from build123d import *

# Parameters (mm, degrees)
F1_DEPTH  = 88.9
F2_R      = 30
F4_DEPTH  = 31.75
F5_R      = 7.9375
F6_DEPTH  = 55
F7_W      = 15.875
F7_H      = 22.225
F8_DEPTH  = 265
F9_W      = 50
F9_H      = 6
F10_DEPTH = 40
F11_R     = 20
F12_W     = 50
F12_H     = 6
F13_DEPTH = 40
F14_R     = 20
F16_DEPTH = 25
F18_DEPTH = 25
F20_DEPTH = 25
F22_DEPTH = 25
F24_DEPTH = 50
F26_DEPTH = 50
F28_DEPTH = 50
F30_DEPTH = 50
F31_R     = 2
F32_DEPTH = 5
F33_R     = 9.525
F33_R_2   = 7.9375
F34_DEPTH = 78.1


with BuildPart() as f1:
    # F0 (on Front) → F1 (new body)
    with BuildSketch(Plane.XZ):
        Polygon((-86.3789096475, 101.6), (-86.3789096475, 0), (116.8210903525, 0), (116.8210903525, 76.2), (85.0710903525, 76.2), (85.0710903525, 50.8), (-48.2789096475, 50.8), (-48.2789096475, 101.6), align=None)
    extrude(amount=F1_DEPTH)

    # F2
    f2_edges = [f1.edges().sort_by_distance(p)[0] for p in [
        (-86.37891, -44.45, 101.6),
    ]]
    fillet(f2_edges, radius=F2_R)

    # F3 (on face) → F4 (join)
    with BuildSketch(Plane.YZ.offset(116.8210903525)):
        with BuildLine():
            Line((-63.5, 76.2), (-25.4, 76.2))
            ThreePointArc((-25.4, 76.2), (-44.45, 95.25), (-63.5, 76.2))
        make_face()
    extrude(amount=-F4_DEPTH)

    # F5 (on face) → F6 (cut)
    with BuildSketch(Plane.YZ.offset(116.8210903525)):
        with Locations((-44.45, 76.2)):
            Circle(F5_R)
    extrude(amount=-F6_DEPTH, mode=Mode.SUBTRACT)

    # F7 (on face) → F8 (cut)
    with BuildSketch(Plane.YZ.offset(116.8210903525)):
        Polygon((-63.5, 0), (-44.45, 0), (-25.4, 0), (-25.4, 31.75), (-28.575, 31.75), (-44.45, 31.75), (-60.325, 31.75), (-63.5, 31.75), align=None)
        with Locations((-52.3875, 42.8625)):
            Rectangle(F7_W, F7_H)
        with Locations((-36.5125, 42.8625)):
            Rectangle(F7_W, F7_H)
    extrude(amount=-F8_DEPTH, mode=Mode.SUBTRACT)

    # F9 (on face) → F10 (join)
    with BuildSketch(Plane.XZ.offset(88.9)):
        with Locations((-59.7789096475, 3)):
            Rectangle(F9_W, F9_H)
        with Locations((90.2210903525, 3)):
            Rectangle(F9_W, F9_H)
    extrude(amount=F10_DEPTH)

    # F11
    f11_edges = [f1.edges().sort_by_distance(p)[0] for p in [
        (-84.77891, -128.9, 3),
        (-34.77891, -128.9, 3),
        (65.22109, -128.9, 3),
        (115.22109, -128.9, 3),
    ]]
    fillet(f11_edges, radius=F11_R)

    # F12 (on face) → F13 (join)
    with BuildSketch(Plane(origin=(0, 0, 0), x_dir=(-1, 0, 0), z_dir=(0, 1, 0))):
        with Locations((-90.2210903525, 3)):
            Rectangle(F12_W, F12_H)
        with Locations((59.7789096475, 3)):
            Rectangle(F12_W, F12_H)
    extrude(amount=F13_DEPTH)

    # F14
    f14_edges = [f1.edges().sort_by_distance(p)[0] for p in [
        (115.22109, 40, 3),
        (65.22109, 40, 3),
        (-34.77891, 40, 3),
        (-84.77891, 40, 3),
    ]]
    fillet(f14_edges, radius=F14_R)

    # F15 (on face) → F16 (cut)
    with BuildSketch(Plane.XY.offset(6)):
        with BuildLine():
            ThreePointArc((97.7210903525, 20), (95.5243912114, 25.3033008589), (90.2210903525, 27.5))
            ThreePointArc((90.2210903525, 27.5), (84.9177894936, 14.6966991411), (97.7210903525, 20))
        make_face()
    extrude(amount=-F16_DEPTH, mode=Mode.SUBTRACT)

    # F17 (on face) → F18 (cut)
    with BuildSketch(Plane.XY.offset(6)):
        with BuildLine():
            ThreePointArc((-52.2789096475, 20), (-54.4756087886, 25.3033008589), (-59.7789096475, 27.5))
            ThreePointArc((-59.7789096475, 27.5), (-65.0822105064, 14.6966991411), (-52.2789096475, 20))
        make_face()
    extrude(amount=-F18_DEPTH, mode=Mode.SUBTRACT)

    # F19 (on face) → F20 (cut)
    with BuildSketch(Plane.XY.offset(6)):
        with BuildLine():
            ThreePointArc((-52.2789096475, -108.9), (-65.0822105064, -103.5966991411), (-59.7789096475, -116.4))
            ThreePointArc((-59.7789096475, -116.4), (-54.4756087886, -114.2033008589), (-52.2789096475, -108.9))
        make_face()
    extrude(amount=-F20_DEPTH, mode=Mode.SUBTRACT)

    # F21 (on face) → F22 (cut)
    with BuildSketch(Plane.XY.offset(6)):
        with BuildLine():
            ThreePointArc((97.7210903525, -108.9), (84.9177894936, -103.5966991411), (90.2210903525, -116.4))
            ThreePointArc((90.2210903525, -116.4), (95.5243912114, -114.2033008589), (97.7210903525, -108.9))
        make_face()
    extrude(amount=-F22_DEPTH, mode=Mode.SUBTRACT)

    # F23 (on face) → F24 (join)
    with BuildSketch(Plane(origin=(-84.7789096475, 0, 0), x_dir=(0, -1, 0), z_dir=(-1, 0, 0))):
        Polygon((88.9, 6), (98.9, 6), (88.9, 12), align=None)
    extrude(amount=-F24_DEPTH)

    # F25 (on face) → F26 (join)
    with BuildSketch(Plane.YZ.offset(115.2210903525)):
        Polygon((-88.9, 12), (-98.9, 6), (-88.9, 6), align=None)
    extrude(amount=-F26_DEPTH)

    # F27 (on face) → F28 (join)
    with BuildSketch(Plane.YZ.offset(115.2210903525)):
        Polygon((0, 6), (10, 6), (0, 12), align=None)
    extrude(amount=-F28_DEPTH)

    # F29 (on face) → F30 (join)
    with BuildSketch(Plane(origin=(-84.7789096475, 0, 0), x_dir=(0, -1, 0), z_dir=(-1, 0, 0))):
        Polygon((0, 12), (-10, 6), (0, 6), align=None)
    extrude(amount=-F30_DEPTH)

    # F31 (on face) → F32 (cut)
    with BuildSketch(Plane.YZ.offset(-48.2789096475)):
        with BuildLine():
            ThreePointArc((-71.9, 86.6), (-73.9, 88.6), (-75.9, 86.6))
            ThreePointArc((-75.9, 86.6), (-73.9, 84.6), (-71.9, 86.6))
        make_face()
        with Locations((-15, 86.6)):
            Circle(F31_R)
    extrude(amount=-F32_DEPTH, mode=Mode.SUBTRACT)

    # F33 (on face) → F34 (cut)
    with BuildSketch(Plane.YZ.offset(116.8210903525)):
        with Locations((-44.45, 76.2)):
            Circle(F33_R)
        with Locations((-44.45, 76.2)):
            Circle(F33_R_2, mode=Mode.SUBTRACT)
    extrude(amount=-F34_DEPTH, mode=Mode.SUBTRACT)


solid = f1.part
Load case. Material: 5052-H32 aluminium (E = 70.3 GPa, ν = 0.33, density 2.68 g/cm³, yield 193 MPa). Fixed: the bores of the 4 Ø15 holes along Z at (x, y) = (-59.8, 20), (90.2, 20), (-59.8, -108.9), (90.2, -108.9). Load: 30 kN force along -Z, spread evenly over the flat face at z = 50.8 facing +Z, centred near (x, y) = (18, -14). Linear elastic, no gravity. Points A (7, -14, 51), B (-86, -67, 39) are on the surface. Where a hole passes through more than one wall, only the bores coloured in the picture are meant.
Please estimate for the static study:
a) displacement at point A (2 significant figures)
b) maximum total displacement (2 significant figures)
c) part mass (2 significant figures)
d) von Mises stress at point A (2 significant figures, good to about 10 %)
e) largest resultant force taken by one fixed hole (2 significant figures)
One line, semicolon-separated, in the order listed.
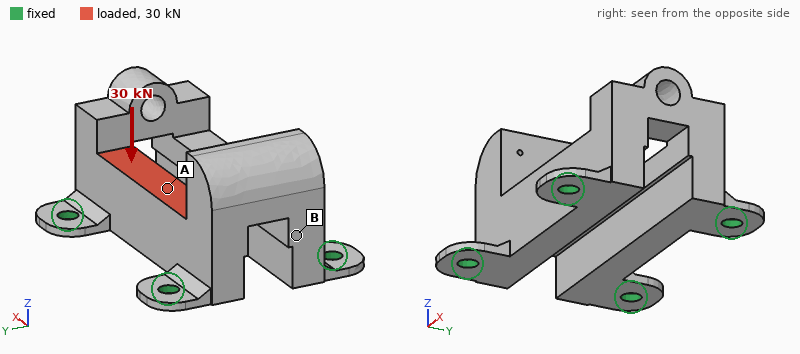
0.17 mm; 0.18 mm; 2.2 kg; 40 MPa; 13 kN
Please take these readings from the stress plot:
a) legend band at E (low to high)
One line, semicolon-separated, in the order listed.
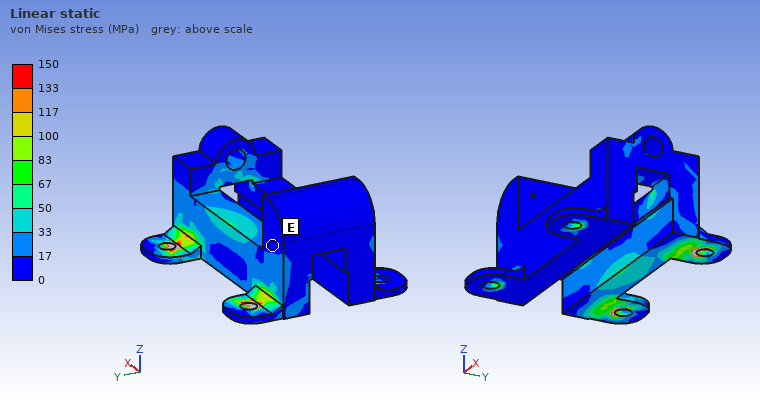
0 to 17 MPa
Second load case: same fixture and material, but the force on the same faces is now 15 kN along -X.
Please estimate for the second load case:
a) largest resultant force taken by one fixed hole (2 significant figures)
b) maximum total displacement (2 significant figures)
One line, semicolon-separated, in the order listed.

7.2 kN; 65 µm
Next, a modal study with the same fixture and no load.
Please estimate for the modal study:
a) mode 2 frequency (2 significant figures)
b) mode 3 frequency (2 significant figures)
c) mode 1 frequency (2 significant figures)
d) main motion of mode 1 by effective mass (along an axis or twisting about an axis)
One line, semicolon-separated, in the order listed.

2300 Hz; 2400 Hz; 2000 Hz; along X
